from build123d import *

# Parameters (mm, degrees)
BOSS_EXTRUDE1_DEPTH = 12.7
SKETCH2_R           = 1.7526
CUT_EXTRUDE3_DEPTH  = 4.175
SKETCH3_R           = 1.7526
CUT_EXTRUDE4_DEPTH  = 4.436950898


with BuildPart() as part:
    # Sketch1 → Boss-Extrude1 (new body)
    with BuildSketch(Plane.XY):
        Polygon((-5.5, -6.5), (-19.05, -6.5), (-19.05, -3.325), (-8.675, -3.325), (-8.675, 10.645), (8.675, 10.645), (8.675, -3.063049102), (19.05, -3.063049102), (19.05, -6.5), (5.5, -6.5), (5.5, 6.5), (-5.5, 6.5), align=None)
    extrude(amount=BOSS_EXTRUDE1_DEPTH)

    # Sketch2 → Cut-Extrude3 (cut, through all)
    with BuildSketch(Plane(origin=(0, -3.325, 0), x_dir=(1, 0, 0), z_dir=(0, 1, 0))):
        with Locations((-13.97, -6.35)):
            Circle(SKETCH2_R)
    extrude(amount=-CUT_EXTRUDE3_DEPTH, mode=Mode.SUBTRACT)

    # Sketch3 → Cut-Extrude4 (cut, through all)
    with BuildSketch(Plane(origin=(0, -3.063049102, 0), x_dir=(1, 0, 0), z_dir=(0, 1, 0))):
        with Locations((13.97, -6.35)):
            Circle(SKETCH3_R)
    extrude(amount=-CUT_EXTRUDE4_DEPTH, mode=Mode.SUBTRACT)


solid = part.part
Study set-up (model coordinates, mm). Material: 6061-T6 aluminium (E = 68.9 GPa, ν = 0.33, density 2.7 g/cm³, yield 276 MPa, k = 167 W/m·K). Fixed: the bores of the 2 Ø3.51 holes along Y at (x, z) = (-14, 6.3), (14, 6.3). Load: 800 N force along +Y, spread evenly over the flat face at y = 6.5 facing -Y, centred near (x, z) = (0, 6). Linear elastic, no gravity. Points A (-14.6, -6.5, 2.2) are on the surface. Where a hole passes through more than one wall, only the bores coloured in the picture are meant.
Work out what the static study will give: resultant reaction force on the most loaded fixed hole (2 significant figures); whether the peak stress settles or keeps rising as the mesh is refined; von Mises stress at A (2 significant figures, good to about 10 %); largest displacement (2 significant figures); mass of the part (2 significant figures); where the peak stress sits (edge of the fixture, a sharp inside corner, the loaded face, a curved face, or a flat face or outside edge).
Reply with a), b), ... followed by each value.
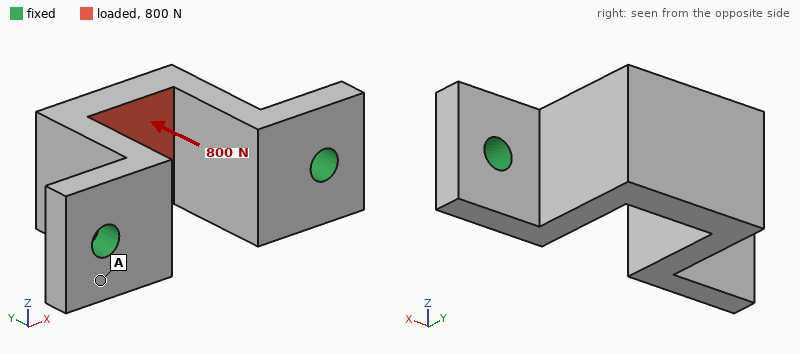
a) 430 N
b) keeps rising
c) 18 MPa
d) 13 µm
e) 7.5 g
f) edge of the fixture
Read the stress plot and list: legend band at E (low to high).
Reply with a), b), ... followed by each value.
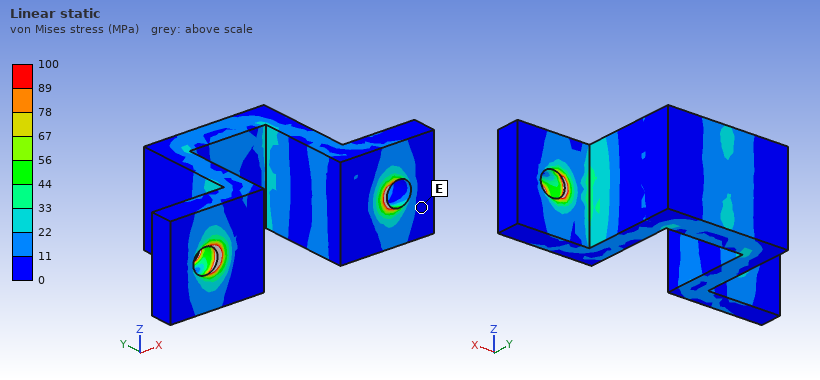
a) 0 to 11 MPa
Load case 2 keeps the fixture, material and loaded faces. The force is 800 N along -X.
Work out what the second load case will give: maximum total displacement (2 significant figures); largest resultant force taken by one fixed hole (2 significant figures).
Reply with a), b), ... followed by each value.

a) 47 µm
b) 520 N
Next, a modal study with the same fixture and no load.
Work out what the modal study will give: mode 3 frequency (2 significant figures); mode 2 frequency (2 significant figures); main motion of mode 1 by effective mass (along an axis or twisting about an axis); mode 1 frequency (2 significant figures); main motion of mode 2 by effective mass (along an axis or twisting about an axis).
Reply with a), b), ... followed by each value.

a) 16 kHz
b) 12 kHz
c) along Z
d) 7200 Hz
e) along X
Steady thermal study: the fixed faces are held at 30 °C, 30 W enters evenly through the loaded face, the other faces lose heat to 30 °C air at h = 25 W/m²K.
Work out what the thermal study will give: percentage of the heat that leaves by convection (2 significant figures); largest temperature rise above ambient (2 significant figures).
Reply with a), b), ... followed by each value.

a) 3.3 %
b) 46 K
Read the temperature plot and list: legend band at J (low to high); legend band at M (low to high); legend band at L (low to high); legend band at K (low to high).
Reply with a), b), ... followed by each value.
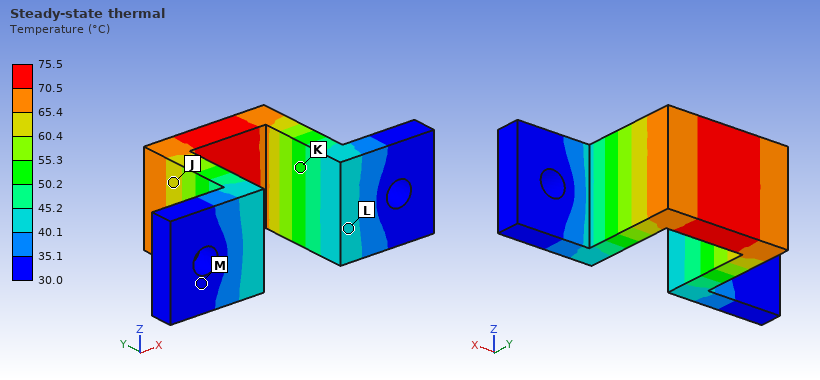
a) 60.4 to 65.4 °C
b) 30.0 to 35.1 °C
c) 40.1 to 45.2 °C
d) 50.2 to 55.3 °C
